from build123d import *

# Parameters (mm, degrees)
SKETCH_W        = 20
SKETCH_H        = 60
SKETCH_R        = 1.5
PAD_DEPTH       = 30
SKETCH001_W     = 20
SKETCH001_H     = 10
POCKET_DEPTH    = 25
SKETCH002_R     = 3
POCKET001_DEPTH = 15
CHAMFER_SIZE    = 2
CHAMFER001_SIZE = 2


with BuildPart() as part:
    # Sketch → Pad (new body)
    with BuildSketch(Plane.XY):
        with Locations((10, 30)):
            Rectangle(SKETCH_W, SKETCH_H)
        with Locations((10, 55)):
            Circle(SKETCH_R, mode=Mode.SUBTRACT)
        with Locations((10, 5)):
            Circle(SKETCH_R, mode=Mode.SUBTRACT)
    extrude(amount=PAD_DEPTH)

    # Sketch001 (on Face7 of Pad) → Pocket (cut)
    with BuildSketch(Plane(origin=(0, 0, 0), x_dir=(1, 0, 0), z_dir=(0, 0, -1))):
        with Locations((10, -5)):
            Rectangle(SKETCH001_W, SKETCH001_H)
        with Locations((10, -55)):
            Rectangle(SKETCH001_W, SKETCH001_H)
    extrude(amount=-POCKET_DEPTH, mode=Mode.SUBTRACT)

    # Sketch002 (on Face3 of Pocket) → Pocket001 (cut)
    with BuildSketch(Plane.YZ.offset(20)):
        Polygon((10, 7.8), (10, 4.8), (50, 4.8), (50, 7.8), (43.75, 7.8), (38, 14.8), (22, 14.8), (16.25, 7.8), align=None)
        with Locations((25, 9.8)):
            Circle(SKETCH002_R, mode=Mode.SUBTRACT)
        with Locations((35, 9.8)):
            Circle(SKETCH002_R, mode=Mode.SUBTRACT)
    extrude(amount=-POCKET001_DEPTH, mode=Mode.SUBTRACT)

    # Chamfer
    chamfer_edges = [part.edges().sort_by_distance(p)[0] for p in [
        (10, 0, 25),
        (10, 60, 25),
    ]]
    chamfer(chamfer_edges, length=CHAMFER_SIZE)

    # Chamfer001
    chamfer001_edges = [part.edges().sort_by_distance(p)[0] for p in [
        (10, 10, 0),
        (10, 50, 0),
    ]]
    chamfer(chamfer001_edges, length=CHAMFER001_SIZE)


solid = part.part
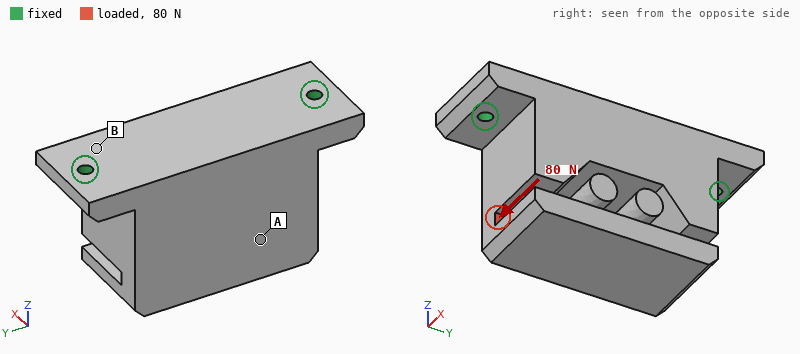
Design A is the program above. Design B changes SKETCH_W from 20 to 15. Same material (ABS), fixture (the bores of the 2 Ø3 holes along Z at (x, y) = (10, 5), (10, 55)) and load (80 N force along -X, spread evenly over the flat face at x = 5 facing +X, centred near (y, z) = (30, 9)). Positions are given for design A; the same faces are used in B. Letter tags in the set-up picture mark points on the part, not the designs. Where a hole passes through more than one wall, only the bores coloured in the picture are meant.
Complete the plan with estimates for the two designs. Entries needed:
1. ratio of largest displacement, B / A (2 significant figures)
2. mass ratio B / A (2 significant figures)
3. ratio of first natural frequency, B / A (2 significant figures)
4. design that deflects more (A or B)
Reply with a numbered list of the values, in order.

1. 1.3
2. 0.74
3. 1.0
4. B
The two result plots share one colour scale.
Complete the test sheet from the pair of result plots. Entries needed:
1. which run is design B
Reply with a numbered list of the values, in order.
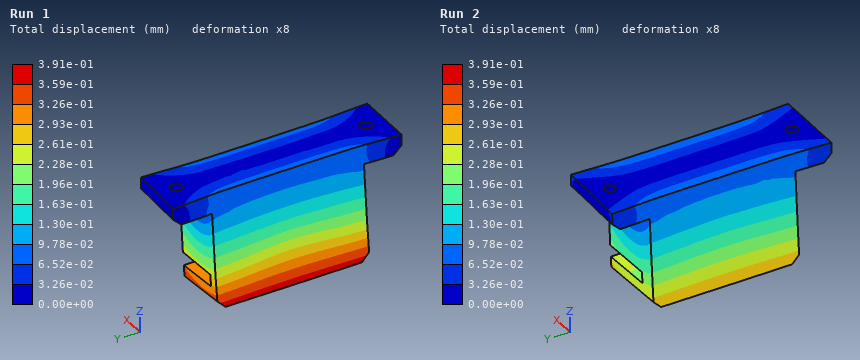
1. Run 1
